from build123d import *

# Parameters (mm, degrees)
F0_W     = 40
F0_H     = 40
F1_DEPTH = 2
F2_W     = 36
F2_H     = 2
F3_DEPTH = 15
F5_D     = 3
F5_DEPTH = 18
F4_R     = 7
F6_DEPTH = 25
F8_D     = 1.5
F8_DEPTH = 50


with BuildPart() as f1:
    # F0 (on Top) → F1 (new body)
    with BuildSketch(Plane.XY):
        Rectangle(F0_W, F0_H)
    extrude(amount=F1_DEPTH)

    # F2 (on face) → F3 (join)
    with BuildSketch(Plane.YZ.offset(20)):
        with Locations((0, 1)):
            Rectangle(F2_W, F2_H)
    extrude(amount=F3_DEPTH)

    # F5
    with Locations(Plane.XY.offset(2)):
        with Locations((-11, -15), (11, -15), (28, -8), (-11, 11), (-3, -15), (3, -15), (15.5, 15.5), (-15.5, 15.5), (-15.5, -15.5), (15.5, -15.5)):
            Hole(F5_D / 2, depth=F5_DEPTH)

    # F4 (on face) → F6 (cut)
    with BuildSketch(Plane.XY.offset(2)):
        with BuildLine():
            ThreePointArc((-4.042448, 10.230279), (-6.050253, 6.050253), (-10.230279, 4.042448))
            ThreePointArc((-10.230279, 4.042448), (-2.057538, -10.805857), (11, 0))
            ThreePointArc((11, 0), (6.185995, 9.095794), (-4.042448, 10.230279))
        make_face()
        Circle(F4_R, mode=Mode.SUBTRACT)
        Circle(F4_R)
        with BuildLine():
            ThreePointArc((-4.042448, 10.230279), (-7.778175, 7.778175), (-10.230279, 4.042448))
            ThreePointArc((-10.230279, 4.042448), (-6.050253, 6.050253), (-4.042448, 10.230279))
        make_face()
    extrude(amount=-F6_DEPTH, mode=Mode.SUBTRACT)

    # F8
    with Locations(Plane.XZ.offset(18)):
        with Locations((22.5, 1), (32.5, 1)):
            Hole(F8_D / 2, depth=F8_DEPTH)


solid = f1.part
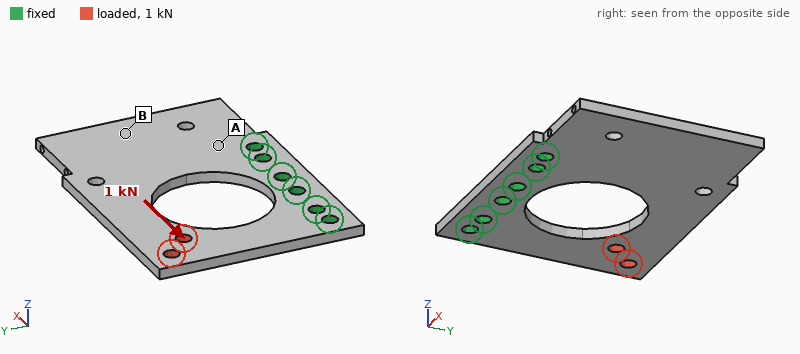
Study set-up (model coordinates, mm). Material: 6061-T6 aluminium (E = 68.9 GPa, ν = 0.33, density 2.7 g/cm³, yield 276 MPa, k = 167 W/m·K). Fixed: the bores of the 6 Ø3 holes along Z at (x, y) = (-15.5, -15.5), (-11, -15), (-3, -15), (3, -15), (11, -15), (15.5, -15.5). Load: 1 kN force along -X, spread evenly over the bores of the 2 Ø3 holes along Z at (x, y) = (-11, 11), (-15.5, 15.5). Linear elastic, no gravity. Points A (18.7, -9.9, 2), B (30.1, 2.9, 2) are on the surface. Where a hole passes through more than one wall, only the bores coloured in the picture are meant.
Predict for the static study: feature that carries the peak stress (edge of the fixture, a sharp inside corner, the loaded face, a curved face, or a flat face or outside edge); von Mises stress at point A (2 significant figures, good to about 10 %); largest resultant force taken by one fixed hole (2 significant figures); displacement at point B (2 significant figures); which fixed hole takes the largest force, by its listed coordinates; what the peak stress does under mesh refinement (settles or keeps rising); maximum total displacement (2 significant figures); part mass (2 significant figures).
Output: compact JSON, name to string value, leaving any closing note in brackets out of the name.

{"feature that carries the peak stress": "edge of the fixture", "von Mises stress at point A": "57 MPa", "largest resultant force taken by one fixed hole": "1.1 kN", "displacement at point B": "60 µm", "which fixed hole takes the largest force, by its listed coordinates": "(15.5, -15.5)", "what the peak stress does under mesh refinement": "keeps rising", "maximum total displacement": "96 µm", "part mass": "8.8 g"}
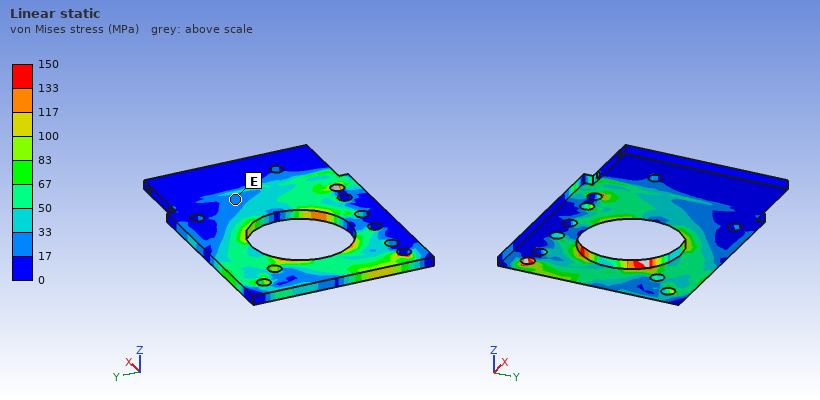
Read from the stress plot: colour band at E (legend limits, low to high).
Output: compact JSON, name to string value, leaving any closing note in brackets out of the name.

{"colour band at E": "17 to 33 MPa"}
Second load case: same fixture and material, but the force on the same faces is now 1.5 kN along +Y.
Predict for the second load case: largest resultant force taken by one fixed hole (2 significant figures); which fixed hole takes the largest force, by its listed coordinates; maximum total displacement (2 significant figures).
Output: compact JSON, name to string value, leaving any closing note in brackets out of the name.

{"largest resultant force taken by one fixed hole": "1.0 kN", "which fixed hole takes the largest force, by its listed coordinates": "(-15.5, -15.5)", "maximum total displacement": "36 µm"}
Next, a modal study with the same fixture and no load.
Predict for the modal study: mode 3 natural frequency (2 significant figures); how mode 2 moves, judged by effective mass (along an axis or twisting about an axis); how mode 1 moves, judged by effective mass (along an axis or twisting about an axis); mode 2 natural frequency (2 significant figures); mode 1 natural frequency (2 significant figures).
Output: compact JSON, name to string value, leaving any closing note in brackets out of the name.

{"mode 3 natural frequency": "4000 Hz", "how mode 2 moves, judged by effective mass": "twisting about Y", "how mode 1 moves, judged by effective mass": "along Z", "mode 2 natural frequency": "1900 Hz", "mode 1 natural frequency": "1100 Hz"}
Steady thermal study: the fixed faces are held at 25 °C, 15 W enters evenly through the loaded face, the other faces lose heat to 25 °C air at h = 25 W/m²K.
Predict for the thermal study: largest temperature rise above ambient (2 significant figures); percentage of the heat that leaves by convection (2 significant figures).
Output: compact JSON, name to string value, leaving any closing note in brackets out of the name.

{"largest temperature rise above ambient": "71 K", "percentage of the heat that leaves by convection": "14 %"}
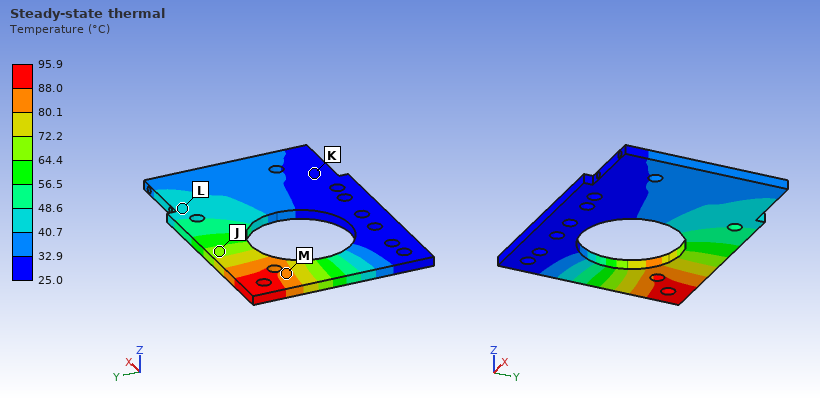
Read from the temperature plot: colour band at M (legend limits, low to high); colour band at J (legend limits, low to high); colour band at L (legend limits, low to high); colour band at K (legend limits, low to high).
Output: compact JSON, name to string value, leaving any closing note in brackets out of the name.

{"colour band at M": "80.1 to 88.0 °C", "colour band at J": "64.4 to 72.2 °C", "colour band at L": "40.7 to 48.6 °C", "colour band at K": "25.0 to 32.9 °C"}
